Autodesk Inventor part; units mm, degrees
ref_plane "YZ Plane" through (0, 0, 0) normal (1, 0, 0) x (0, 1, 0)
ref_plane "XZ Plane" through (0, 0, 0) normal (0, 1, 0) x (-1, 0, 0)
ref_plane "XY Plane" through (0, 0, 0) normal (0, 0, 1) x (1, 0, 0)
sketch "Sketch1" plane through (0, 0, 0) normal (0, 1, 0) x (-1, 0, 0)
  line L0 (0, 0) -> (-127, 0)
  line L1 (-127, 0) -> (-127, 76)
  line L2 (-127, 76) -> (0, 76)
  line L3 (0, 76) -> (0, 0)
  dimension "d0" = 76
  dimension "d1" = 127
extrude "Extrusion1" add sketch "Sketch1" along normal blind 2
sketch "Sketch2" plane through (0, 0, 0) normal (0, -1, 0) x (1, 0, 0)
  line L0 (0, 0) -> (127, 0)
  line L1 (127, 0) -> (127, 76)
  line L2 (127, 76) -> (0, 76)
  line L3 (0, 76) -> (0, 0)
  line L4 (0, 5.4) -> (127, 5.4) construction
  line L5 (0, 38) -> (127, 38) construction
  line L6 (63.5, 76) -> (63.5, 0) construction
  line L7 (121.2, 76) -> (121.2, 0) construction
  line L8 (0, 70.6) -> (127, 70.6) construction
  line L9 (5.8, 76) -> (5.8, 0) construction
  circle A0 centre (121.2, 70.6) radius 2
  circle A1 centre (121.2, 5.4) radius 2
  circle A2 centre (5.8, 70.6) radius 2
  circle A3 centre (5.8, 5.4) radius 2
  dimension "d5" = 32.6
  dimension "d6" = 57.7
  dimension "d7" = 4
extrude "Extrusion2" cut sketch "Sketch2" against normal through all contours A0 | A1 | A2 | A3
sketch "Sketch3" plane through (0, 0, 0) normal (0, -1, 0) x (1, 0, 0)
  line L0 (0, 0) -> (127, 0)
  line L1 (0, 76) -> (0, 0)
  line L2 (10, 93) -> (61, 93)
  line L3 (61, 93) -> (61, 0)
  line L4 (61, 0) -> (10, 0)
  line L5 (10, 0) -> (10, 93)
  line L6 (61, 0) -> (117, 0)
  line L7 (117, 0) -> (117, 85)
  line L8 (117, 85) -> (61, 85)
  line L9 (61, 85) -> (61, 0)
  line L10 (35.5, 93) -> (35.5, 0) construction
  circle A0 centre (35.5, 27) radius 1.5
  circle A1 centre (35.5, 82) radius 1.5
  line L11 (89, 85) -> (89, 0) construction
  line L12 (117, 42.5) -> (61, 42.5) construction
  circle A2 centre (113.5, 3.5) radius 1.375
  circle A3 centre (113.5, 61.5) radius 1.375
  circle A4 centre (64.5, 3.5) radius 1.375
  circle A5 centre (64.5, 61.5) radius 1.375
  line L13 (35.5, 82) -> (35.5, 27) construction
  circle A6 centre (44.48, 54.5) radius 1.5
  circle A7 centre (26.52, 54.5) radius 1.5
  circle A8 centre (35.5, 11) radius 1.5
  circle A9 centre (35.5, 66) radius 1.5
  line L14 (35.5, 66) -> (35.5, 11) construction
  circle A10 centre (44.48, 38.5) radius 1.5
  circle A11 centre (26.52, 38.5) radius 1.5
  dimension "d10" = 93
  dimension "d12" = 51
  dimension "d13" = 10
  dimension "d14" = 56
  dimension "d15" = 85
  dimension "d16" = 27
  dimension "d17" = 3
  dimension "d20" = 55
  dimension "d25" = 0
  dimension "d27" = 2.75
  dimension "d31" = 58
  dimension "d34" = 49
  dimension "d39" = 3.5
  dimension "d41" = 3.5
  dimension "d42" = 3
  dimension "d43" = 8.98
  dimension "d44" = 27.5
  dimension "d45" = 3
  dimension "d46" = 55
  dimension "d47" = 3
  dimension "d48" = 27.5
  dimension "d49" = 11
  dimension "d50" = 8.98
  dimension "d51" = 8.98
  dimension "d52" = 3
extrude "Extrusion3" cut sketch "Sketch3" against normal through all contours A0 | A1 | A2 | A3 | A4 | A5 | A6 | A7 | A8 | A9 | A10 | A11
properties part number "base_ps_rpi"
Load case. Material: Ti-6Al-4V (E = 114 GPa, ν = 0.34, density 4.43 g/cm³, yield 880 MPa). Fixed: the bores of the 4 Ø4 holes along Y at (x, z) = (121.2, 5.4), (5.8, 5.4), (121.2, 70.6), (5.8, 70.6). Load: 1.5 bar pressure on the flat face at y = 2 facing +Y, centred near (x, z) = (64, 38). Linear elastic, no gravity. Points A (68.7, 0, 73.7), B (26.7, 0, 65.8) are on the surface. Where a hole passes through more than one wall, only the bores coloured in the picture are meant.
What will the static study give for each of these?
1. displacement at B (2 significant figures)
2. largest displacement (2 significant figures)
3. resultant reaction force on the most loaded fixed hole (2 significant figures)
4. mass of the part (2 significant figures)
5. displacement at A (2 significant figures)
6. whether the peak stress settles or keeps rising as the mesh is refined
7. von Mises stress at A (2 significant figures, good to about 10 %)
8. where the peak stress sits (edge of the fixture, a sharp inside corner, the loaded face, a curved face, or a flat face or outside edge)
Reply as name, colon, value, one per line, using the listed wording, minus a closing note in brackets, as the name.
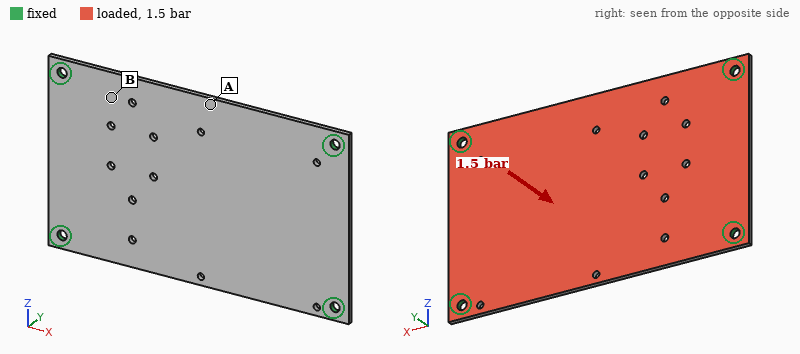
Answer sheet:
displacement at B: 0.49 mm
largest displacement: 1.3 mm
resultant reaction force on the most loaded fixed hole: 360 N
mass of the part: 84 g
displacement at A: 1.2 mm
whether the peak stress settles or keeps rising as the mesh is refined: keeps rising
von Mises stress at A: 160 MPa
where the peak stress sits: edge of the fixture
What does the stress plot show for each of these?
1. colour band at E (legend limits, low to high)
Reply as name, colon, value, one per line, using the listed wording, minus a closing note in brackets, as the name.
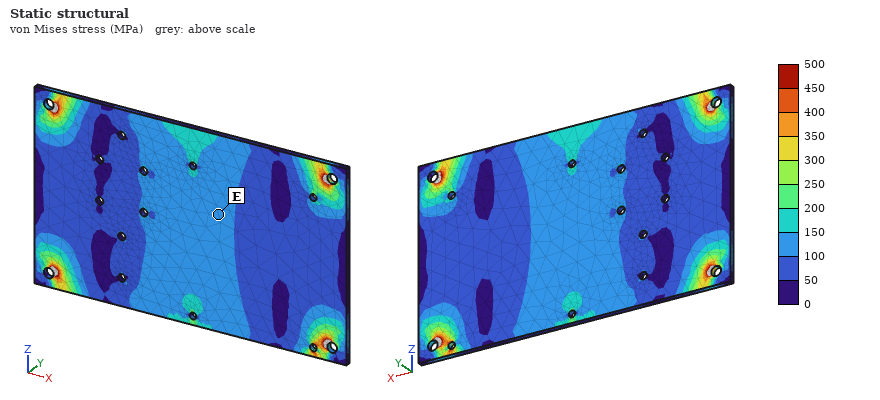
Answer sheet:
colour band at E: 100 to 150 MPa
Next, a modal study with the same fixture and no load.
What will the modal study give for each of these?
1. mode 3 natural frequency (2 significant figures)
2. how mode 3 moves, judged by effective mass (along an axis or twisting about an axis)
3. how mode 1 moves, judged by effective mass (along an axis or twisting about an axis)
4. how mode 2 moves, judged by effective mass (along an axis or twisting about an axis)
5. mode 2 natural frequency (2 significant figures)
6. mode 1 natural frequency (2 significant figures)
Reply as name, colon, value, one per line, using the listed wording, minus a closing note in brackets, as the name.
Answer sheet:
mode 3 natural frequency: 1800 Hz
how mode 3 moves, judged by effective mass: twisting about Z
how mode 1 moves, judged by effective mass: along Y
how mode 2 moves, judged by effective mass: twisting about X
mode 2 natural frequency: 1100 Hz
mode 1 natural frequency: 670 Hz
